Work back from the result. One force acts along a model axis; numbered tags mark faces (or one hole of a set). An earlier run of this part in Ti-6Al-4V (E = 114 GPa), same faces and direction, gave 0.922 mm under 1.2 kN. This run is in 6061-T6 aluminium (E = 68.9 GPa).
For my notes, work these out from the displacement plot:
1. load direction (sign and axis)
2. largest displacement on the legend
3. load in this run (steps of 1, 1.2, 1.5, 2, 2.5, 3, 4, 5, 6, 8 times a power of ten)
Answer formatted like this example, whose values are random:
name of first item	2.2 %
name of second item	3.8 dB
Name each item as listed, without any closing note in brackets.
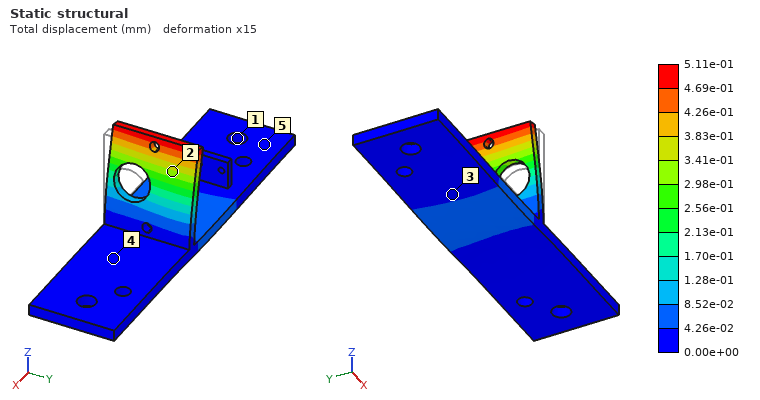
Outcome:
load direction	-X
largest displacement on the legend	5.11e-01 mm
load in this run	400 N
